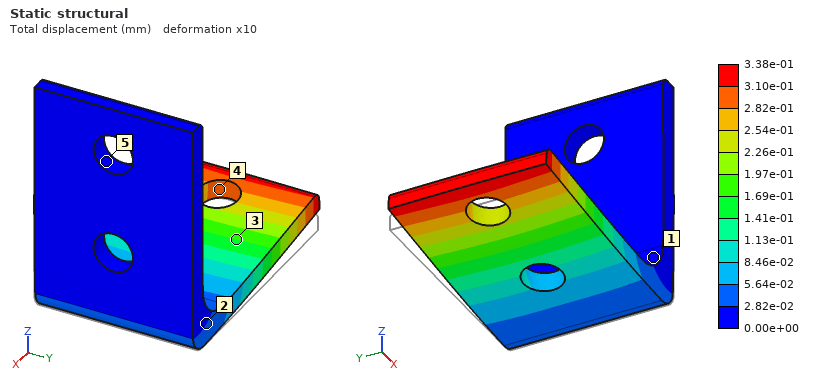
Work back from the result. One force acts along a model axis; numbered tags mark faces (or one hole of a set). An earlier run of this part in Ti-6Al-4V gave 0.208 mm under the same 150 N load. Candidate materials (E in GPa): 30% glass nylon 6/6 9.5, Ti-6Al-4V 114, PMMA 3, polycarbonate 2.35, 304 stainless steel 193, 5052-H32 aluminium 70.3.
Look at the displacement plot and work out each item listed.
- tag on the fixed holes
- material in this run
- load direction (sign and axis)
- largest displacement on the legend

5
5052-H32 aluminium
+Z
3.38e-01 mm
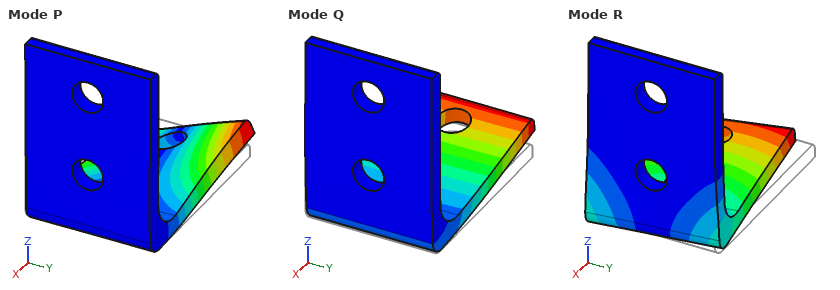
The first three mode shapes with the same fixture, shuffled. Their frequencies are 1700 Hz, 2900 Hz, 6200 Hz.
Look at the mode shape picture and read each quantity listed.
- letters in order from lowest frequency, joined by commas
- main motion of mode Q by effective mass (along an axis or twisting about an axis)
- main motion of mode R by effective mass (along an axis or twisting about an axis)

Q, R, P
along Z
along Y
